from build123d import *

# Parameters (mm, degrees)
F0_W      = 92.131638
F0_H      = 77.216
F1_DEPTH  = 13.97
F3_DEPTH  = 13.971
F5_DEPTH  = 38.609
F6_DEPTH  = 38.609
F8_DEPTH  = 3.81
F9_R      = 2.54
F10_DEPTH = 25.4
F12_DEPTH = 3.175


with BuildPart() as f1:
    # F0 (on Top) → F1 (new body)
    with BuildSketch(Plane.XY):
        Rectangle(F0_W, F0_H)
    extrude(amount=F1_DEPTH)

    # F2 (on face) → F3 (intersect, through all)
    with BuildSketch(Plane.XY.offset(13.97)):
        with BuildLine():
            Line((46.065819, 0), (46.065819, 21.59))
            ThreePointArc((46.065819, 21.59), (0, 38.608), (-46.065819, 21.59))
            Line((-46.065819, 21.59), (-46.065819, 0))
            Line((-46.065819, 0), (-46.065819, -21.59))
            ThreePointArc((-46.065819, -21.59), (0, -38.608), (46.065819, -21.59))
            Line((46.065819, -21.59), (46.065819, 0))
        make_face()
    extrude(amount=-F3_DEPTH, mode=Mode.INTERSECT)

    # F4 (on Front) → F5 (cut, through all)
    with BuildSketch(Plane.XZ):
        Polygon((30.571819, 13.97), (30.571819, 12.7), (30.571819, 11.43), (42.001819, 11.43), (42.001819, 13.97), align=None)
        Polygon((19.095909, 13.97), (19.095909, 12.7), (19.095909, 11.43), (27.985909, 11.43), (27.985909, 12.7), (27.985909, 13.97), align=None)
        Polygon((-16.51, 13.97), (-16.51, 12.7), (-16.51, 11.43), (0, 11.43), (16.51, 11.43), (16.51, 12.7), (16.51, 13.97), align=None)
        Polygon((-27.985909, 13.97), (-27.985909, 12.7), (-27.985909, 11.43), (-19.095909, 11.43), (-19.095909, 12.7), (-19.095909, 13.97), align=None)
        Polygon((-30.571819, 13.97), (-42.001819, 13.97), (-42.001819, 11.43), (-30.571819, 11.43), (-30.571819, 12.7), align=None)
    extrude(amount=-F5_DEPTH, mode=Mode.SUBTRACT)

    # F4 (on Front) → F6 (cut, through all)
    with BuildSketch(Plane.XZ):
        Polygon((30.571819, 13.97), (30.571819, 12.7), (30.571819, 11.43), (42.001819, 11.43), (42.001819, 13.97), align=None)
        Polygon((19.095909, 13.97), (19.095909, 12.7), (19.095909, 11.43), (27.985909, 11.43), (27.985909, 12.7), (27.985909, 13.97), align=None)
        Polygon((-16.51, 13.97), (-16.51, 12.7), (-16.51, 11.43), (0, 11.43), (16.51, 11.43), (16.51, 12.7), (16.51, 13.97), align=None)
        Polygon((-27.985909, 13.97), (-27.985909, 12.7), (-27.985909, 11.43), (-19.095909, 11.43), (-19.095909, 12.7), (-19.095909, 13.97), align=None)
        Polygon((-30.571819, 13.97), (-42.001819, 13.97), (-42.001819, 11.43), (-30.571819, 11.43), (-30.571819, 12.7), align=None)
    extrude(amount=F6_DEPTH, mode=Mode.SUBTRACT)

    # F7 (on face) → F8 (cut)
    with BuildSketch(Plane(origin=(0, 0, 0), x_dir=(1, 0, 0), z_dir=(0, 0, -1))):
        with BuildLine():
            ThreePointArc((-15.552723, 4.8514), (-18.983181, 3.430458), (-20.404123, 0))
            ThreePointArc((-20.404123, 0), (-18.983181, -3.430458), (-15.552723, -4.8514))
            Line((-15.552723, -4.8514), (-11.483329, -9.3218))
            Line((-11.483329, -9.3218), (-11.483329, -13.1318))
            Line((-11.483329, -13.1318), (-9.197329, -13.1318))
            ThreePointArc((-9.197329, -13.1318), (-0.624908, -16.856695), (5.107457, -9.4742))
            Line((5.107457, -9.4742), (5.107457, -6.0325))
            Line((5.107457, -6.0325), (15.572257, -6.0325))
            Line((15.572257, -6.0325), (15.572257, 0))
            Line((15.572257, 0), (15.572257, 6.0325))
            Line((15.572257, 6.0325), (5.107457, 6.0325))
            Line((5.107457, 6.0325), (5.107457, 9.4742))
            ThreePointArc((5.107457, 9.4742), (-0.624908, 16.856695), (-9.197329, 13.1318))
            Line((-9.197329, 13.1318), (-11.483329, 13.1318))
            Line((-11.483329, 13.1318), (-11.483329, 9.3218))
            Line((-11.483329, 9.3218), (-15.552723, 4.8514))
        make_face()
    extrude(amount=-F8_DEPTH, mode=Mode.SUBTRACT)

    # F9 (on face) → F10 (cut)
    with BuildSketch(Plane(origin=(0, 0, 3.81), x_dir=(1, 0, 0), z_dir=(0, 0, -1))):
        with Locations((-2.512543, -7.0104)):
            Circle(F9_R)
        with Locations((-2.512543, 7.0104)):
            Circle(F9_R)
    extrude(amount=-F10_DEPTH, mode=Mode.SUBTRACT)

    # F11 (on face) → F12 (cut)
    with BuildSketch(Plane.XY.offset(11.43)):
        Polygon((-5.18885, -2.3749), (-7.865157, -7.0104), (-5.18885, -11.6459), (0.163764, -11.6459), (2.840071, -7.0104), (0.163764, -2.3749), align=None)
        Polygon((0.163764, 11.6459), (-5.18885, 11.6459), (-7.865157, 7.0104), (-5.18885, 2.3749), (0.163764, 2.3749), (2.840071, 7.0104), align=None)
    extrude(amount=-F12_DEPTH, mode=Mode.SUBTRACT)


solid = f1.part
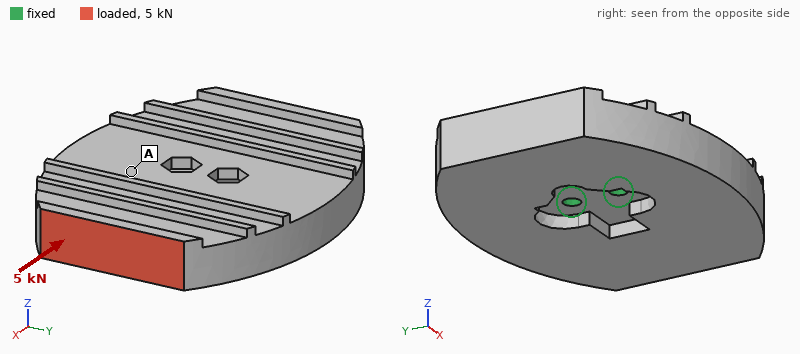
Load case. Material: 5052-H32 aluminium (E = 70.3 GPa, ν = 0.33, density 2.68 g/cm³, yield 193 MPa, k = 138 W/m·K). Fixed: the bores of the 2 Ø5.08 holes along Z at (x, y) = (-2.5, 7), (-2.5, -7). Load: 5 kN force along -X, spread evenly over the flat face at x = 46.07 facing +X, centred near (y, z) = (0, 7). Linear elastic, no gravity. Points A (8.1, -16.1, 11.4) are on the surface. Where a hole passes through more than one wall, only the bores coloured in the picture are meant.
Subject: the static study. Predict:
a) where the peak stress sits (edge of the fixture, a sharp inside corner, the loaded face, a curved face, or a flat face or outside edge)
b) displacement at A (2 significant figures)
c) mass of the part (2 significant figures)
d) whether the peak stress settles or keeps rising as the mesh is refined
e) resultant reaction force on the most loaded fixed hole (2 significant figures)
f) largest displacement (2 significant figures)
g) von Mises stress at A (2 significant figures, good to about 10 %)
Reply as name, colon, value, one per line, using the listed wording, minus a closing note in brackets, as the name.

where the peak stress sits: edge of the fixture
displacement at A: 7.9 µm
mass of the part: 190 g
whether the peak stress settles or keeps rising as the mesh is refined: keeps rising
resultant reaction force on the most loaded fixed hole: 2.5 kN
largest displacement: 33 µm
von Mises stress at A: 8.8 MPa
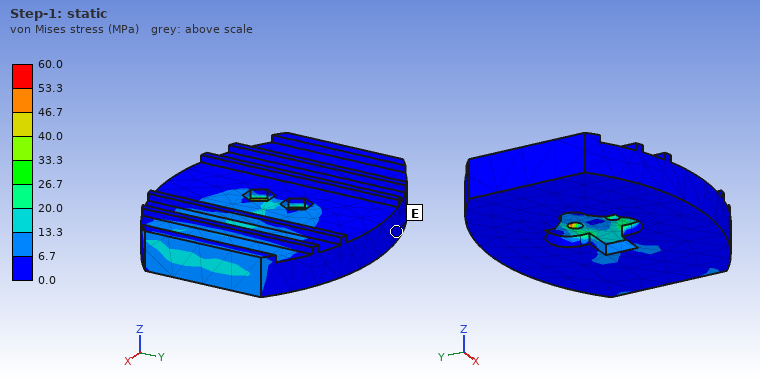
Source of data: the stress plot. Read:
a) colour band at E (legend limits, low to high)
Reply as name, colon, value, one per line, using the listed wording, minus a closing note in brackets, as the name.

colour band at E: 0.0 to 6.7 MPa
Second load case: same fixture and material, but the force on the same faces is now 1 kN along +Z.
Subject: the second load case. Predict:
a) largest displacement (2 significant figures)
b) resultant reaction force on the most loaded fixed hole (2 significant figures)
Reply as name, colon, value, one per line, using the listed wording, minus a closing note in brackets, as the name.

largest displacement: 0.30 mm
resultant reaction force on the most loaded fixed hole: 500 N
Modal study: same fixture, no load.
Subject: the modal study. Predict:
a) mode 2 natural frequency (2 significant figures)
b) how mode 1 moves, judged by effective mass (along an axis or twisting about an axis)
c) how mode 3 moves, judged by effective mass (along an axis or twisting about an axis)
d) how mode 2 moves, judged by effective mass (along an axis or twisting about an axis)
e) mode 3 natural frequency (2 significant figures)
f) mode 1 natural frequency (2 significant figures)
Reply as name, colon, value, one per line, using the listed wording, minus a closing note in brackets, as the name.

mode 2 natural frequency: 3100 Hz
how mode 1 moves, judged by effective mass: twisting about Y
how mode 3 moves, judged by effective mass: twisting about Z
how mode 2 moves, judged by effective mass: twisting about X
mode 3 natural frequency: 3400 Hz
mode 1 natural frequency: 1400 Hz
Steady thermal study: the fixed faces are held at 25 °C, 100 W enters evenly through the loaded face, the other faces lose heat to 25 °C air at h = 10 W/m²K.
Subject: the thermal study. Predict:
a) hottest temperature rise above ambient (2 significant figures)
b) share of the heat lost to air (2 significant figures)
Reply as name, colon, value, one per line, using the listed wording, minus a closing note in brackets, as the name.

hottest temperature rise above ambient: 69 K
share of the heat lost to air: 4.6 %
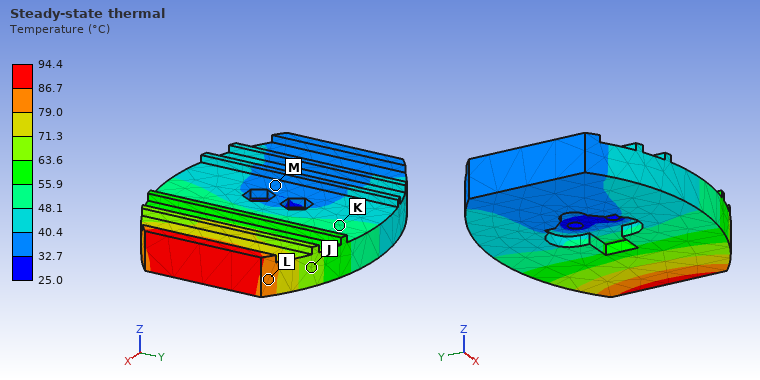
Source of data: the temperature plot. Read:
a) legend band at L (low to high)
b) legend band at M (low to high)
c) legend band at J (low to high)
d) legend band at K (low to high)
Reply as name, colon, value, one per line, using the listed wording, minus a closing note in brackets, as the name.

legend band at L: 79.0 to 86.7 °C
legend band at M: 32.7 to 40.4 °C
legend band at J: 63.6 to 71.3 °C
legend band at K: 48.1 to 55.9 °C
